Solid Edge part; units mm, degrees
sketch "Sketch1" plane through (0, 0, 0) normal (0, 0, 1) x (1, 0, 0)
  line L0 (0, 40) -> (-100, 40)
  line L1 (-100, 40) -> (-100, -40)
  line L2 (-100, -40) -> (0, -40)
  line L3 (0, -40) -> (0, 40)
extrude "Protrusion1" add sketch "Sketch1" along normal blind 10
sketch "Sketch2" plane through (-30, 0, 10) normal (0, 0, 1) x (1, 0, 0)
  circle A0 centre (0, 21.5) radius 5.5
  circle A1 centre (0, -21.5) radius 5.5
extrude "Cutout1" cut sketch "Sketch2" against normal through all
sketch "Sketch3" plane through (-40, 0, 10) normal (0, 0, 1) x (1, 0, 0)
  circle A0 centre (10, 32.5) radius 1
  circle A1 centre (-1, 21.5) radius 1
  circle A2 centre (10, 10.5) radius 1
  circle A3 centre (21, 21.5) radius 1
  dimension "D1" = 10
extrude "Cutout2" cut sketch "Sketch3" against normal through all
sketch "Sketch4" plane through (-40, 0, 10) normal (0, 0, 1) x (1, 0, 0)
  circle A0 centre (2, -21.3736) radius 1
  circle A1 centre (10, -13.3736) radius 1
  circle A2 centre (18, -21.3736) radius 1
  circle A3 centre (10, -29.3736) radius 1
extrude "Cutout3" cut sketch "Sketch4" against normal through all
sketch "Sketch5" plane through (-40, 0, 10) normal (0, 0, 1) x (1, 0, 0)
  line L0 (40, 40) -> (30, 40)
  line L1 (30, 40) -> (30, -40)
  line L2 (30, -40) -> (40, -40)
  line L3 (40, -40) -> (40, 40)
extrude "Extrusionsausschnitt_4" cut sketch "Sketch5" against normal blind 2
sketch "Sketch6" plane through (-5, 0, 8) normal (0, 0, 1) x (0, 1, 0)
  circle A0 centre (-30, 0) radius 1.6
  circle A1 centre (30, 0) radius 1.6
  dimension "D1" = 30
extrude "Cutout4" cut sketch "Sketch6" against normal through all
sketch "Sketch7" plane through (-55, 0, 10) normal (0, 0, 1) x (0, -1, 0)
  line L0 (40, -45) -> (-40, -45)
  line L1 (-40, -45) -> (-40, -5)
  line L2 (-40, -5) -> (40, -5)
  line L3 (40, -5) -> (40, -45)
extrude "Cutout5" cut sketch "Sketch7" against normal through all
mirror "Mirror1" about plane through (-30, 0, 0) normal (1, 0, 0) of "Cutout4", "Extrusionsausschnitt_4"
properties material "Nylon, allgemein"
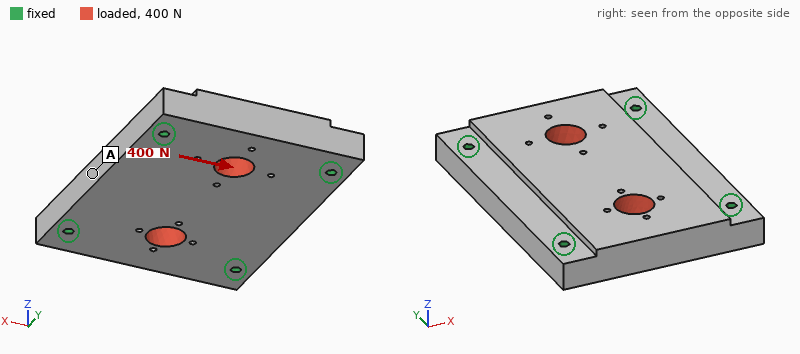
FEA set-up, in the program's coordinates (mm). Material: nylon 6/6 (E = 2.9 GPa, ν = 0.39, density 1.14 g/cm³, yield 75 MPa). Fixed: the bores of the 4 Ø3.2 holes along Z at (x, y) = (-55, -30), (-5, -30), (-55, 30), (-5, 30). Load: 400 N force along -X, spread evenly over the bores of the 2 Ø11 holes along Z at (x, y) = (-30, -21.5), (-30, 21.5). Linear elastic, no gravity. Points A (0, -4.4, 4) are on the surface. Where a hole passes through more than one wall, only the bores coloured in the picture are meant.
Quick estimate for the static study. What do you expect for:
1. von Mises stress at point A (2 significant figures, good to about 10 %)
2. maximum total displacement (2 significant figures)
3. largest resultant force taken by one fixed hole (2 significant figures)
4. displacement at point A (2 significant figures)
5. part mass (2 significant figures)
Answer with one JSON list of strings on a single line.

["0.23 MPa", "8.6 µm", "110 N", "7.1 µm", "48 g"]
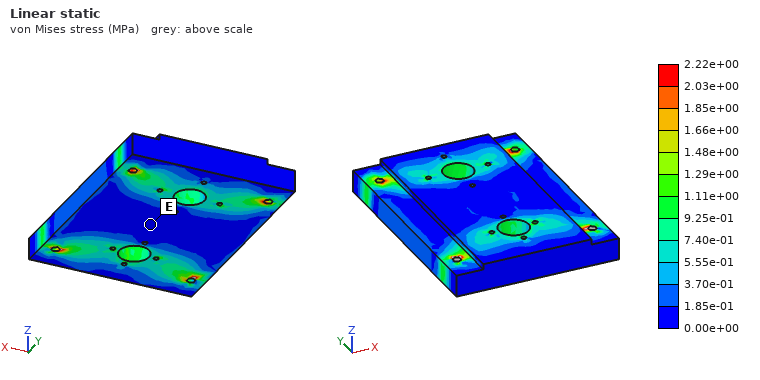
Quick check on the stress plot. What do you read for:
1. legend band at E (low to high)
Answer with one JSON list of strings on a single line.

["0.00e+00 to 1.85e-01 MPa"]
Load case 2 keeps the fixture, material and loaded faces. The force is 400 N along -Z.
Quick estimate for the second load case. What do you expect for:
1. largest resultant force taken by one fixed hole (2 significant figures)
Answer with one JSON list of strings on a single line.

["110 N"]
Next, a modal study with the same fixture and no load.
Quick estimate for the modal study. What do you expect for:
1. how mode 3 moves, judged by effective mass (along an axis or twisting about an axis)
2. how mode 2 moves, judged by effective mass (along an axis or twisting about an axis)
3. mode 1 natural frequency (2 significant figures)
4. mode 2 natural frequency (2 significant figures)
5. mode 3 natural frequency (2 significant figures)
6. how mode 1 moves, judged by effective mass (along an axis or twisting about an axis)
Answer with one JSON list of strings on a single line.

["twisting about X", "twisting about Y", "2500 Hz", "3800 Hz", "4300 Hz", "along Z"]
